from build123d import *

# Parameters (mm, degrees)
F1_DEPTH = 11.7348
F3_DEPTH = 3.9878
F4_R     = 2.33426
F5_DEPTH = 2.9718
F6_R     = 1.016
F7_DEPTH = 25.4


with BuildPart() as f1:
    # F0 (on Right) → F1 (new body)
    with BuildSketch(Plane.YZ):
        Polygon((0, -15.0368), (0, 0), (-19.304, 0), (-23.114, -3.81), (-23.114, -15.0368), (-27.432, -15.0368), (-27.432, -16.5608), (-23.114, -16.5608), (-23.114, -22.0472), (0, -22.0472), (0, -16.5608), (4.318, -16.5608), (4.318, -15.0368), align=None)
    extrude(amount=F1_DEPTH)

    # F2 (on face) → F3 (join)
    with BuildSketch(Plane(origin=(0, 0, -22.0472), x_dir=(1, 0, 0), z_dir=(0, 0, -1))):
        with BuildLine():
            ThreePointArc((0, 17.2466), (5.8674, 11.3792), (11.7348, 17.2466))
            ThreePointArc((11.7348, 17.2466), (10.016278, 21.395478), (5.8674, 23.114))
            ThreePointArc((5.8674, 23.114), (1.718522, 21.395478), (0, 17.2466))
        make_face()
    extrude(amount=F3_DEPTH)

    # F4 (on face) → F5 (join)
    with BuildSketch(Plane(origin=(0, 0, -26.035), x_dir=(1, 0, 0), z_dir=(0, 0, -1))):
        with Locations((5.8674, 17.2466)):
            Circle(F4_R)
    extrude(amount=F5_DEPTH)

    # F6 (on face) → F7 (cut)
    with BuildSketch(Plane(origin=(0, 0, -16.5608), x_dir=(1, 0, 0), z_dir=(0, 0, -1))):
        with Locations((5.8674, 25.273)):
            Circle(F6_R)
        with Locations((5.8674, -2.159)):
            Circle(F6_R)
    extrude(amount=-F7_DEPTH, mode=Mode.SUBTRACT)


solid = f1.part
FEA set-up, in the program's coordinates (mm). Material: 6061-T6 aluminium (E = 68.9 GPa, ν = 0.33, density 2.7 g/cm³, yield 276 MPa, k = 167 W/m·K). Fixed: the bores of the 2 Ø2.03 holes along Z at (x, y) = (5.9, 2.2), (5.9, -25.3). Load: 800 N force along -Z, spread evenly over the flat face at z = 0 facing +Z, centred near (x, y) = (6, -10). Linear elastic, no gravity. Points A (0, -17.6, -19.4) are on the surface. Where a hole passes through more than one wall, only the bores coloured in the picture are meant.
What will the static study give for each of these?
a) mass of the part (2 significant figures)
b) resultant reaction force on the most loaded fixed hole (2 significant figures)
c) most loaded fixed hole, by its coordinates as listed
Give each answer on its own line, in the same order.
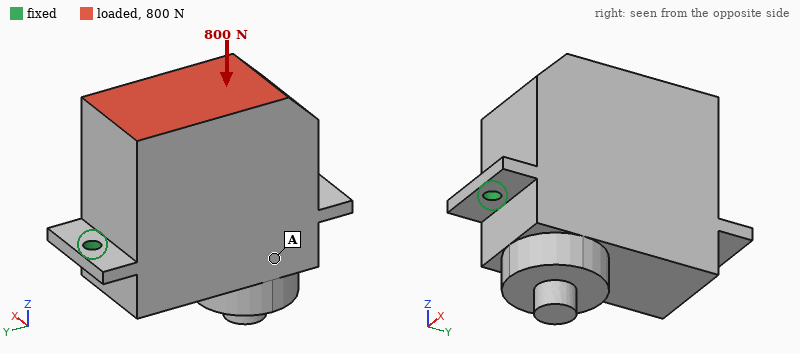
18 g
460 N
(5.9, 2.2)
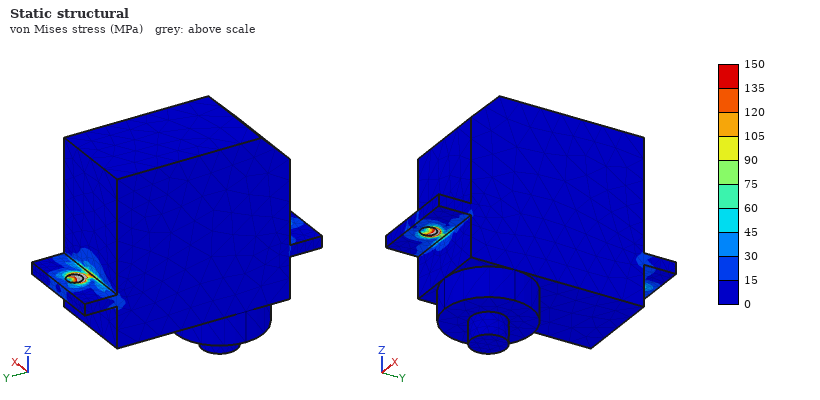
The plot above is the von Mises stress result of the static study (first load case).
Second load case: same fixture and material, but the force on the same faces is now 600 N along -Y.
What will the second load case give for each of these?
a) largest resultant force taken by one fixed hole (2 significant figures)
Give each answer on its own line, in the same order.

490 N
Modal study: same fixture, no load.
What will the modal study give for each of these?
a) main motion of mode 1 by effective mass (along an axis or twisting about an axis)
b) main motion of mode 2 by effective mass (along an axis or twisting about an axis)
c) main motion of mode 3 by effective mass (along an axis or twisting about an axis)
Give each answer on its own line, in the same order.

along X
along Z
along Y
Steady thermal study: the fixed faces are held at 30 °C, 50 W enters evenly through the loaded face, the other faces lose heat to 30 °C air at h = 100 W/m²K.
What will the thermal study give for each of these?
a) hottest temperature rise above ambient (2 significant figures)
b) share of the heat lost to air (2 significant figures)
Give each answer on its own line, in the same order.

50 K
15 %
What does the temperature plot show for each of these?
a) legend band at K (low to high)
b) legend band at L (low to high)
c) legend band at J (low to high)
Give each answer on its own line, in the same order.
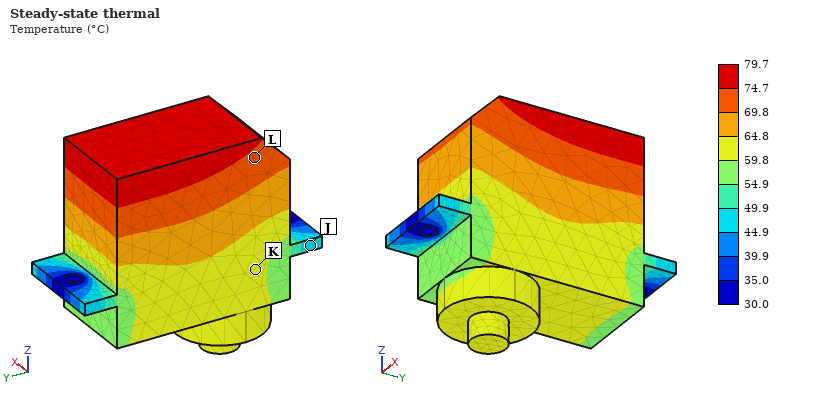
59.8 to 64.8 °C
69.8 to 74.7 °C
44.9 to 49.9 °C
